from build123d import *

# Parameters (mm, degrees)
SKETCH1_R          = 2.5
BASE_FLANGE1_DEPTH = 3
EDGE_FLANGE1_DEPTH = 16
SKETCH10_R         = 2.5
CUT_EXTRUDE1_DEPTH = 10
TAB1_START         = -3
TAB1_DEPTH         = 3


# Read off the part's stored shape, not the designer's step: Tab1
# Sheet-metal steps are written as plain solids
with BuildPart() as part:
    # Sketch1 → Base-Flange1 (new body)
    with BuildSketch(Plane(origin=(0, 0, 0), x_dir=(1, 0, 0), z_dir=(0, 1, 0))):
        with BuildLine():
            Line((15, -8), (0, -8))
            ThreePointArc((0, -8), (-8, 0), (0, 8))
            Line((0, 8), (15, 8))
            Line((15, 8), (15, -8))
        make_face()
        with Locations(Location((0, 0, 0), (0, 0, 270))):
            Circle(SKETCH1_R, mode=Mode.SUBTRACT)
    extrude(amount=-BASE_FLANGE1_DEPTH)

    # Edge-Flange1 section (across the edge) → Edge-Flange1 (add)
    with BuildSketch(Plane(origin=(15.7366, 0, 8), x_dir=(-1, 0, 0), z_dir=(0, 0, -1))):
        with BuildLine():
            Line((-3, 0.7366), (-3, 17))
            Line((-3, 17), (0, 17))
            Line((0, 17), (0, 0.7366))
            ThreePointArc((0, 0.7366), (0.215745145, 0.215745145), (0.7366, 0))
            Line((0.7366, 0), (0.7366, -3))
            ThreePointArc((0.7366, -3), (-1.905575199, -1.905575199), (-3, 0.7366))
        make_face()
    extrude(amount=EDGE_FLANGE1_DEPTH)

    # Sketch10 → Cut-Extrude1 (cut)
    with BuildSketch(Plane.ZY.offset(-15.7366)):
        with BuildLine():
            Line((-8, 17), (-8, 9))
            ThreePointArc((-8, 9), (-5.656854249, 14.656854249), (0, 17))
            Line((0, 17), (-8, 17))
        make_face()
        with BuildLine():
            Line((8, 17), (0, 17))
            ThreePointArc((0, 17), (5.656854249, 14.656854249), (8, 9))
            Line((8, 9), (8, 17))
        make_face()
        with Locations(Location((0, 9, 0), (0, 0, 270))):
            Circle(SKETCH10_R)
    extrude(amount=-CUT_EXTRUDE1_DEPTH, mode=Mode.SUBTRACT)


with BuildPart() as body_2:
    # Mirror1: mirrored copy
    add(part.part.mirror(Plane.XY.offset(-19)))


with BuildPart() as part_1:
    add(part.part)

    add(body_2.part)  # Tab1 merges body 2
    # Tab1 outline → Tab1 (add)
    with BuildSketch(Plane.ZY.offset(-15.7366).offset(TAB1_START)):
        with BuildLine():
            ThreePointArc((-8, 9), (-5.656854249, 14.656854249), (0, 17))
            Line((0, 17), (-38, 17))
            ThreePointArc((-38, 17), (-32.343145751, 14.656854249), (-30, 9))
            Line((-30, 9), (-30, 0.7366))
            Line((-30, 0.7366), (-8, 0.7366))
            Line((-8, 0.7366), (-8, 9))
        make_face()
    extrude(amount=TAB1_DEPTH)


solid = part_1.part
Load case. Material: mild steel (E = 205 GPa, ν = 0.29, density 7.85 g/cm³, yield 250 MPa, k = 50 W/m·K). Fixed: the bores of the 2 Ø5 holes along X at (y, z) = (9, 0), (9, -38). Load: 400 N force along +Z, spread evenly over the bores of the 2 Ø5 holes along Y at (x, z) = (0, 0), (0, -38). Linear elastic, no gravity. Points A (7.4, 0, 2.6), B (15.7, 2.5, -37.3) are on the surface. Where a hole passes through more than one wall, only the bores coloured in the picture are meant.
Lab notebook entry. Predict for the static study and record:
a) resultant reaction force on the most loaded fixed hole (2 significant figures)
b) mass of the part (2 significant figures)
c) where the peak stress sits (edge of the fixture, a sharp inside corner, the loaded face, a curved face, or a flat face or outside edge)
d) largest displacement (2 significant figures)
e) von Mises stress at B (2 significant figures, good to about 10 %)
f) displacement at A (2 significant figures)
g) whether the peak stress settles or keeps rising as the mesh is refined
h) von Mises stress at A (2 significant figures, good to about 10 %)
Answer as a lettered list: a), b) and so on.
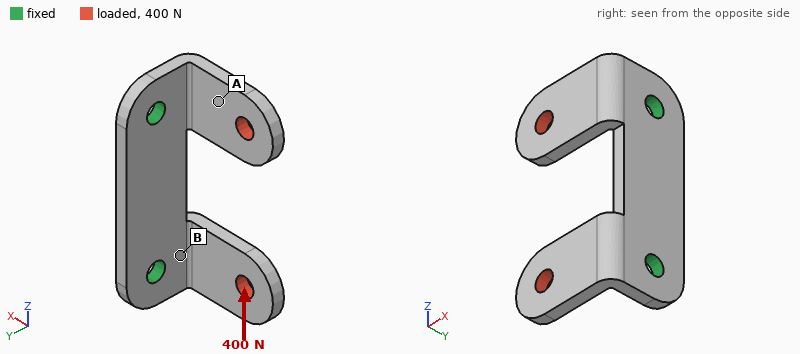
a) 220 N
b) 37 g
c) a sharp inside corner
d) 46 µm
e) 81 MPa
f) 19 µm
g) keeps rising
h) 16 MPa
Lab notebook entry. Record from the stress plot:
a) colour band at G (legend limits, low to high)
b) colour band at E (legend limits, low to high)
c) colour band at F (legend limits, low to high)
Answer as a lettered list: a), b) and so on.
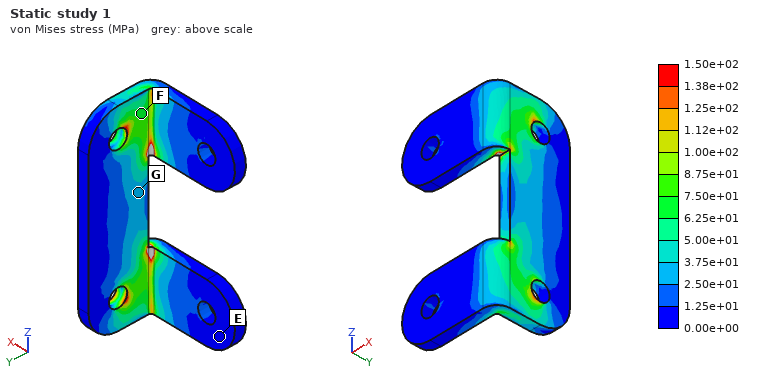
a) 2.50e+01 to 3.75e+01 MPa
b) 0.00e+00 to 1.25e+01 MPa
c) 6.25e+01 to 7.50e+01 MPa
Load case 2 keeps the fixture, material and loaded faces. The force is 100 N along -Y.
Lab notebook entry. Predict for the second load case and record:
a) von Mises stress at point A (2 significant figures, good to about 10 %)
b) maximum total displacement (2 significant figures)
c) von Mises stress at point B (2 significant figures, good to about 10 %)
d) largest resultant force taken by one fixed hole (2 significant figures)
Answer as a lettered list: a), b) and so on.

a) 15 MPa
b) 42 µm
c) 33 MPa
d) 50 N
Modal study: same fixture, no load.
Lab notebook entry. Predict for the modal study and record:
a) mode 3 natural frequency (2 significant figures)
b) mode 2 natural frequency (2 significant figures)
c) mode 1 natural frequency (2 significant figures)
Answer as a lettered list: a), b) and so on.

a) 4800 Hz
b) 3000 Hz
c) 3000 Hz
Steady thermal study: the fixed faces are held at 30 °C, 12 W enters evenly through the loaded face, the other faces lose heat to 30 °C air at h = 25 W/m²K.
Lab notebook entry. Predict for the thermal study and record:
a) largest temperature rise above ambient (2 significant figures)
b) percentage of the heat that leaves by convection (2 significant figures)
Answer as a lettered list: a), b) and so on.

a) 62 K
b) 18 %
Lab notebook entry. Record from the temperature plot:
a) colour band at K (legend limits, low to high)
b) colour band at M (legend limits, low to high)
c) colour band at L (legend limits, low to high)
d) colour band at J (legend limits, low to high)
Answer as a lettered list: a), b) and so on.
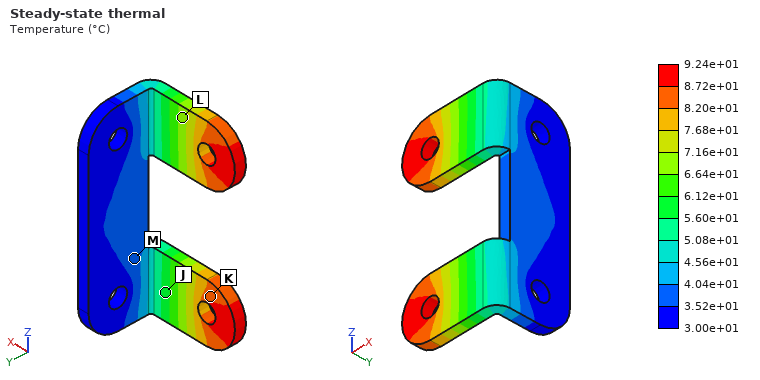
a) 8.20e+01 to 8.72e+01 °C
b) 3.52e+01 to 4.04e+01 °C
c) 6.64e+01 to 7.16e+01 °C
d) 5.60e+01 to 6.12e+01 °C
